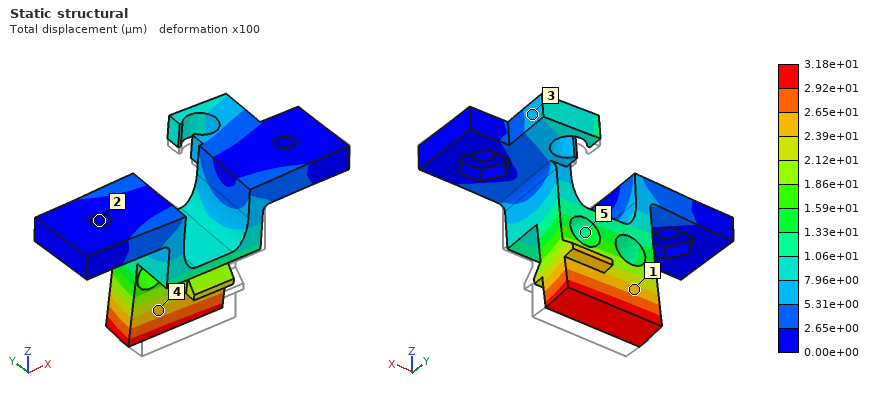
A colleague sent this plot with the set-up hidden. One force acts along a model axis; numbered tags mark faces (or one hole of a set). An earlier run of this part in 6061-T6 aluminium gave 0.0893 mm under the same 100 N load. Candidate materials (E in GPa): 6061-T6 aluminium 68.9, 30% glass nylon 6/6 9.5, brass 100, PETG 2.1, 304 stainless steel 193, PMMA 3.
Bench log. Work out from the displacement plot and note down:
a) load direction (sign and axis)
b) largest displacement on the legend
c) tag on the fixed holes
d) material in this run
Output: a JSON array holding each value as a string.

["+Y", "3.18e+01 µm", "2", "304 stainless steel"]
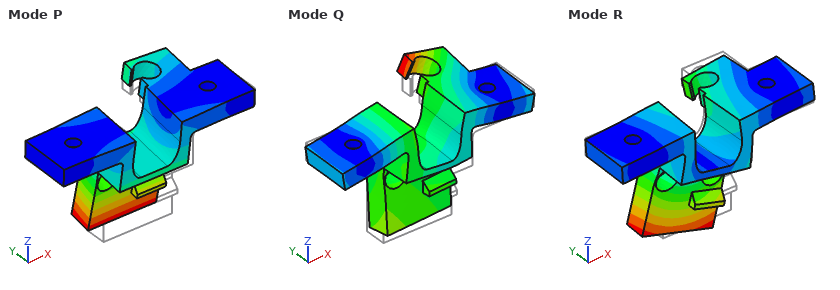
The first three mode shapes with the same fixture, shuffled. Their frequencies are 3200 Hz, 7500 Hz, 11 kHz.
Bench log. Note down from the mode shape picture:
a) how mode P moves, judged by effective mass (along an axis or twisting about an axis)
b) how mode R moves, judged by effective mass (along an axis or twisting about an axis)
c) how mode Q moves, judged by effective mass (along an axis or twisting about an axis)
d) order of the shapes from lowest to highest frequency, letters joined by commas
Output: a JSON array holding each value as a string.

["along Y", "along X", "along Z", "P, R, Q"]
